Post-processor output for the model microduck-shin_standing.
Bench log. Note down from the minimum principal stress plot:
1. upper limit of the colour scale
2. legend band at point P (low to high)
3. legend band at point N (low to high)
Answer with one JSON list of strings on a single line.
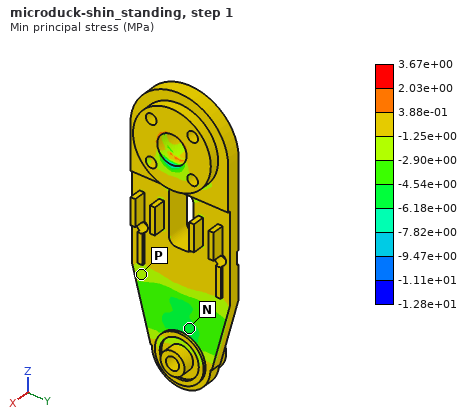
["3.67e+00 MPa", "-2.90e+00 to -1.25e+00 MPa", "-6.18e+00 to -4.54e+00 MPa"]
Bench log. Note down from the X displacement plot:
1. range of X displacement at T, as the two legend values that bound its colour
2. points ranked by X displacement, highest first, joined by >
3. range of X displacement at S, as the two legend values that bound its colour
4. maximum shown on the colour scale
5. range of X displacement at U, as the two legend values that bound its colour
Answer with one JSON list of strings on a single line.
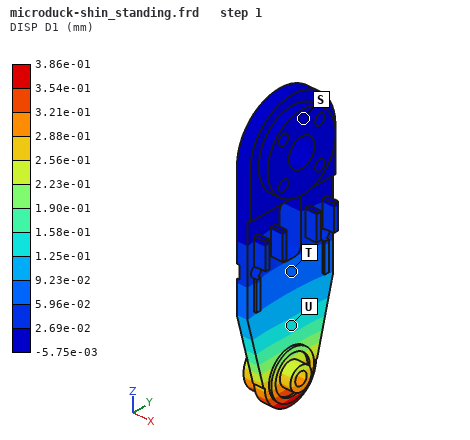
["5.96e-02 to 9.23e-02 mm", "U > T > S", "-5.75e-03 to 2.69e-02 mm", "3.86e-01 mm", "1.25e-01 to 1.58e-01 mm"]
